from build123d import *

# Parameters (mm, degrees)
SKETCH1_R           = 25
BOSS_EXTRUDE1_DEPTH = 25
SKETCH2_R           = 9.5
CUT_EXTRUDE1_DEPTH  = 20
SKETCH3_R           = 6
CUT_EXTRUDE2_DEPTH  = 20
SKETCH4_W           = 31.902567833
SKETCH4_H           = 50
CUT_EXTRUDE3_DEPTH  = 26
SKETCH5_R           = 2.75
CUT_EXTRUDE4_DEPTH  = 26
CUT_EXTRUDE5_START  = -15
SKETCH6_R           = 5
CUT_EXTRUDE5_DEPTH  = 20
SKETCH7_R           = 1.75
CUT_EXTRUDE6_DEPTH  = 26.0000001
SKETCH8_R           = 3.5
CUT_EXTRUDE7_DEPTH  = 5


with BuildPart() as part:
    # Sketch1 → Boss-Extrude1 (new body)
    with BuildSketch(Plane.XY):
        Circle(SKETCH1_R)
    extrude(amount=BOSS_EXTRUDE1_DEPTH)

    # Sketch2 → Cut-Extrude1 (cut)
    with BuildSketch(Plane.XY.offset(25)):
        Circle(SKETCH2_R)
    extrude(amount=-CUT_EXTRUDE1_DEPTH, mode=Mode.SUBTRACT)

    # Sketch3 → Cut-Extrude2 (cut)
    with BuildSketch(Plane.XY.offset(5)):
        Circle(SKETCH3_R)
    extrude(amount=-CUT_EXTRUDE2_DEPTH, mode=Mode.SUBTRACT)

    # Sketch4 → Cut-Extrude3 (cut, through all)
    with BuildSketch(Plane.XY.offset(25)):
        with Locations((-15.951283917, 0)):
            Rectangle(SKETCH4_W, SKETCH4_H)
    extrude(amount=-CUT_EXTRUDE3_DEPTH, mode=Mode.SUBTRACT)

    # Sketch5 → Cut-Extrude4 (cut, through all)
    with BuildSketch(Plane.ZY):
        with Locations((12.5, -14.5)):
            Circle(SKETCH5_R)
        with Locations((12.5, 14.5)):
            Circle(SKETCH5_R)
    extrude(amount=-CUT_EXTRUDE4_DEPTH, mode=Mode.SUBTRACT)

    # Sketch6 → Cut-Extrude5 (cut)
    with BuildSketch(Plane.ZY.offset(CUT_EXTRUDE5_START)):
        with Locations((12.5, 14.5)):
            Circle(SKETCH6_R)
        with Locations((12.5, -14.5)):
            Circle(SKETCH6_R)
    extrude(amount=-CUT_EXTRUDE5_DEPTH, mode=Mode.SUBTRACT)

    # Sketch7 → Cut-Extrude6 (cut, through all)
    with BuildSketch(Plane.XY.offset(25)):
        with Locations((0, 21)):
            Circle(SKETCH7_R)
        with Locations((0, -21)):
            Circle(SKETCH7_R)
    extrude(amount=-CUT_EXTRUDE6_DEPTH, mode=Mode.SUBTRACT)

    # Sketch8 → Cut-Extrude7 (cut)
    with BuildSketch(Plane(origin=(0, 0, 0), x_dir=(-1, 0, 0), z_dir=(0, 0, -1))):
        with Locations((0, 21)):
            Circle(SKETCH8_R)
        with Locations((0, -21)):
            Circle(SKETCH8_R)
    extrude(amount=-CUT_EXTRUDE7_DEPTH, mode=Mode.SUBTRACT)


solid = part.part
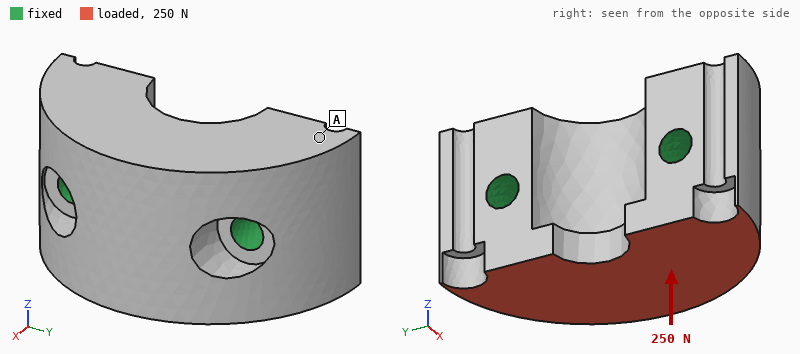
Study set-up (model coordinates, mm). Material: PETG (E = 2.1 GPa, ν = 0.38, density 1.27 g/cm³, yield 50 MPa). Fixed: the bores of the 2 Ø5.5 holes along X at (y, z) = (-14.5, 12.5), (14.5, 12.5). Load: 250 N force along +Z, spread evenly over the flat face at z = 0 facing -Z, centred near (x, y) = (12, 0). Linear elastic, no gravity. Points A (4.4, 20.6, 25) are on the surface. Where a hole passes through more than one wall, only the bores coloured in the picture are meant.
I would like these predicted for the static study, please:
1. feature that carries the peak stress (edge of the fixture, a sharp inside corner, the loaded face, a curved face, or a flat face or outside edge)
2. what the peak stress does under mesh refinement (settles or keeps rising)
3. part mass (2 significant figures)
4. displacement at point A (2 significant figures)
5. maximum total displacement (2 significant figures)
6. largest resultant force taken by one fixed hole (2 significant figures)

edge of the fixture
keeps rising
25 g
1.8 µm
11 µm
130 N
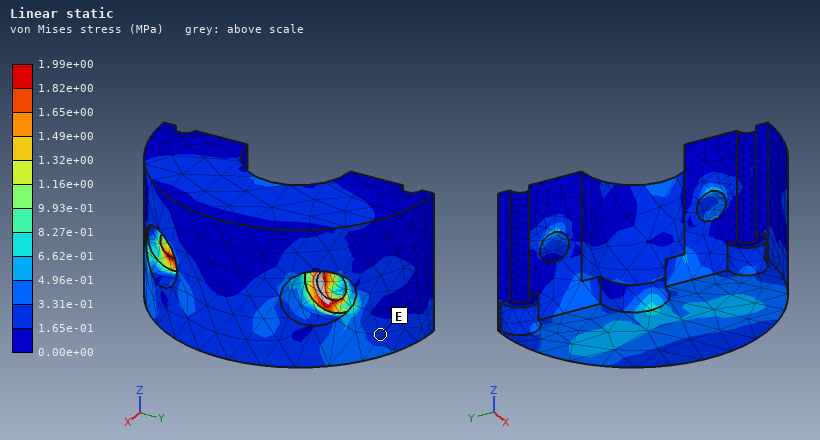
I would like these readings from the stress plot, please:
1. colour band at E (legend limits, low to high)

1.65e-01 to 3.31e-01 MPa
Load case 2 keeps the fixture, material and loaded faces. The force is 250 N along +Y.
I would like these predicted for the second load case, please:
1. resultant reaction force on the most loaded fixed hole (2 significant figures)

150 N
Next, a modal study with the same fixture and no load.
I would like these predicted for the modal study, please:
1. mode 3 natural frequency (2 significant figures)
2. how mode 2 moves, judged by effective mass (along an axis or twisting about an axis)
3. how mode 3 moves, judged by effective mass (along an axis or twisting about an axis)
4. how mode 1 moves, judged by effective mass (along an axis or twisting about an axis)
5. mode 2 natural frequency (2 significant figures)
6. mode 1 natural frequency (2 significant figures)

9500 Hz
along X
twisting about X
along Z
8900 Hz
5600 Hz
